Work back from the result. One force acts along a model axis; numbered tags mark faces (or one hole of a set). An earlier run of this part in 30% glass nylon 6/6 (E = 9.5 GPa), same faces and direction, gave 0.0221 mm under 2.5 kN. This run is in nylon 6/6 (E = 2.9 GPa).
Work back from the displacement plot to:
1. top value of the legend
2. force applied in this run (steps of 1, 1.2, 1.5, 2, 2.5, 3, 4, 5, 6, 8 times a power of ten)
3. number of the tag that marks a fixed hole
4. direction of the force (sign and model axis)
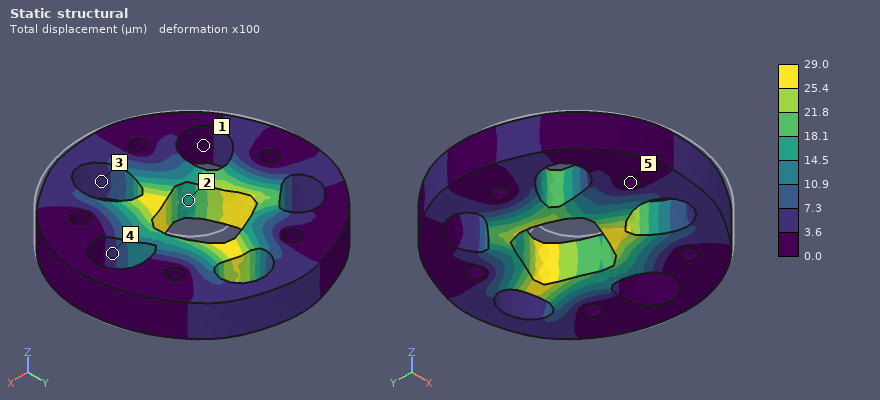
29.0 µm
1 kN
5
+Y
